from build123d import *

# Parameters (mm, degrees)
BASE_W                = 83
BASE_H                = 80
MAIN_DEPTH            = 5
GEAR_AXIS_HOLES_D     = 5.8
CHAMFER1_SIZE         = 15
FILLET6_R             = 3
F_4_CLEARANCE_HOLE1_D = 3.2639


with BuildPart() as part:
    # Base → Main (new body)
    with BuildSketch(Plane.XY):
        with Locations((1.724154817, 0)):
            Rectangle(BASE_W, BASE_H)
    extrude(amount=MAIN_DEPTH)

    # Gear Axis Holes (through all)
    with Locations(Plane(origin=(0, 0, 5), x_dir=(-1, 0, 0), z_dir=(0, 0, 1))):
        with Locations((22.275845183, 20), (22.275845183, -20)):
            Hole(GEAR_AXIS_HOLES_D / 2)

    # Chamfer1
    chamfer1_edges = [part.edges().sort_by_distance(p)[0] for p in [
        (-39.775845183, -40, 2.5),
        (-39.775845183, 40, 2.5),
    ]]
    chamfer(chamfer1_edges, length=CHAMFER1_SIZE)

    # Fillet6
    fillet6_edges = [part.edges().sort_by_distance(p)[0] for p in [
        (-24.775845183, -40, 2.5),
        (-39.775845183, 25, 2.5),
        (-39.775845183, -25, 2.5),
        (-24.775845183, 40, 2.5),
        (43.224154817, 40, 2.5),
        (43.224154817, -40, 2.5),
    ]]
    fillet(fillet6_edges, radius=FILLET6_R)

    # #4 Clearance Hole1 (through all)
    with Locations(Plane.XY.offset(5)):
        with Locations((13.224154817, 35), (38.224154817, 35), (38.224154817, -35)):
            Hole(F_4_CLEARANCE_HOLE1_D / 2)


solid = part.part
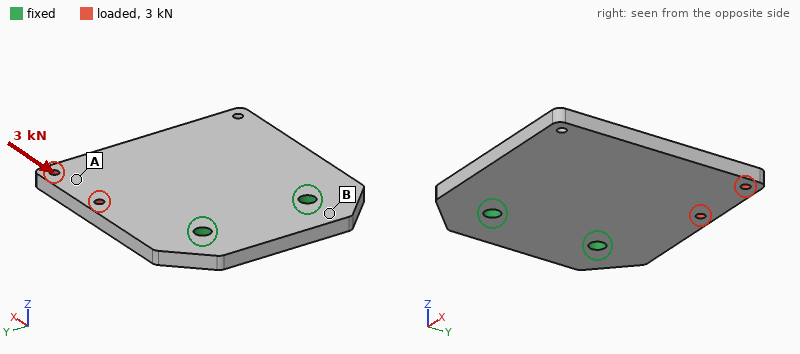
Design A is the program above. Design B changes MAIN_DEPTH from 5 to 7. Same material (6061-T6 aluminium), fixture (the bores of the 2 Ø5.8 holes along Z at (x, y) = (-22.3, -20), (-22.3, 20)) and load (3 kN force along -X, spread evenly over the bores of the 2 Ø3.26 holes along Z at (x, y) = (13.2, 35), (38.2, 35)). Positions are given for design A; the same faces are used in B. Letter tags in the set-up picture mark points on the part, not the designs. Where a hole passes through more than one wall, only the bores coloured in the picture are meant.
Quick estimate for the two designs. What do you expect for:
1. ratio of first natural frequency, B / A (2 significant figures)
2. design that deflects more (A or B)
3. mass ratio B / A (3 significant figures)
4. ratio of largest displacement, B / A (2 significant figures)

1.4
A
1.40
0.71
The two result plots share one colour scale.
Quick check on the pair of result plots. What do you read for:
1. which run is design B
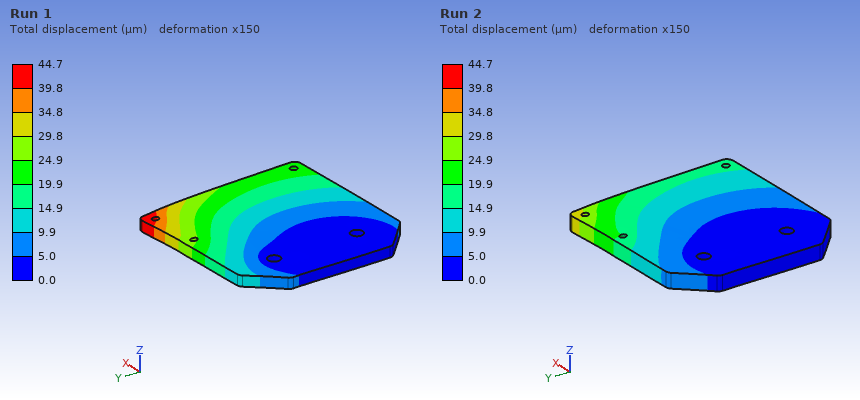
Run 2
